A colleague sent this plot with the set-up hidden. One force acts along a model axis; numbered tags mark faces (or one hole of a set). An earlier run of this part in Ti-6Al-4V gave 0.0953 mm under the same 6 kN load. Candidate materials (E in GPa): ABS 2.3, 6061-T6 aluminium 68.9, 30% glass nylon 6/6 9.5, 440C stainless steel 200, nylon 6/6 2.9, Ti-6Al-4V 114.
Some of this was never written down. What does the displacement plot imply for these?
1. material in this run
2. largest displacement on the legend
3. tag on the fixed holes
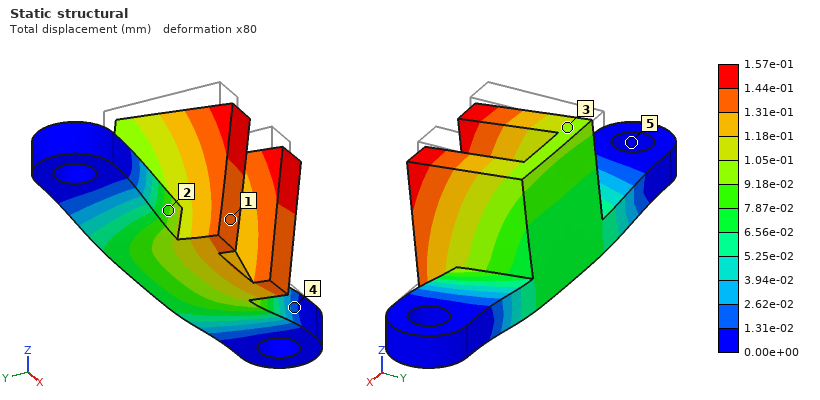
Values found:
6061-T6 aluminium
1.57e-01 mm
5
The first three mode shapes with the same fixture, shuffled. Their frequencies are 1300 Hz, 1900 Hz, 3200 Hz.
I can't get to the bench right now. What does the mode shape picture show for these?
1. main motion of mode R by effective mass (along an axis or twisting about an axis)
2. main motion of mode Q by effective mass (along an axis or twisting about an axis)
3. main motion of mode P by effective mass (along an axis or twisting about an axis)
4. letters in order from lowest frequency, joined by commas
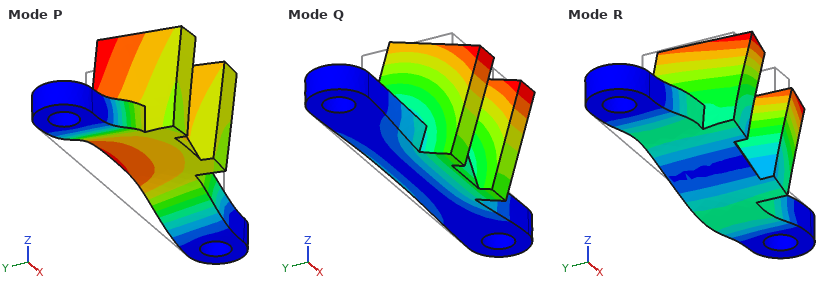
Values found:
along X
along Y
along Z
Q, P, R
